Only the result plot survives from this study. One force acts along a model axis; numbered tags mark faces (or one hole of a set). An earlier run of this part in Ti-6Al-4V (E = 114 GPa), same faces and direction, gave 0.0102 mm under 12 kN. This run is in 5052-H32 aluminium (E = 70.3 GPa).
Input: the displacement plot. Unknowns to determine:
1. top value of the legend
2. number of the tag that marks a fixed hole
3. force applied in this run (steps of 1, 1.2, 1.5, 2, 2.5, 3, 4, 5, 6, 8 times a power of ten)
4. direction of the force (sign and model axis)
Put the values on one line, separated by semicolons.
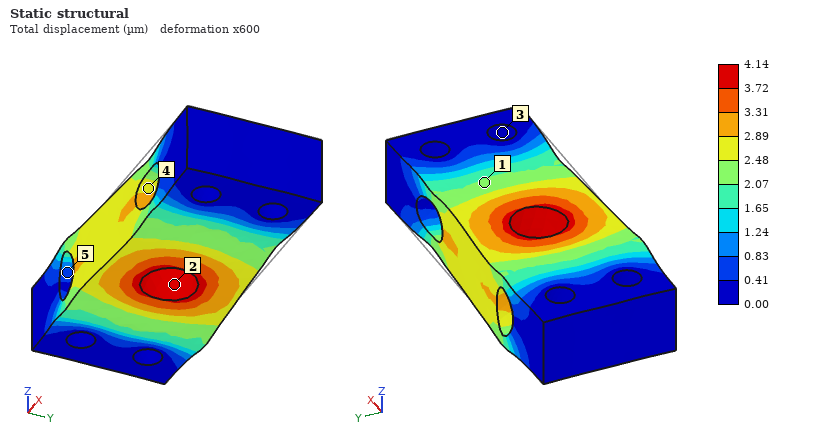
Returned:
4.14 µm; 3; 3 kN; -X
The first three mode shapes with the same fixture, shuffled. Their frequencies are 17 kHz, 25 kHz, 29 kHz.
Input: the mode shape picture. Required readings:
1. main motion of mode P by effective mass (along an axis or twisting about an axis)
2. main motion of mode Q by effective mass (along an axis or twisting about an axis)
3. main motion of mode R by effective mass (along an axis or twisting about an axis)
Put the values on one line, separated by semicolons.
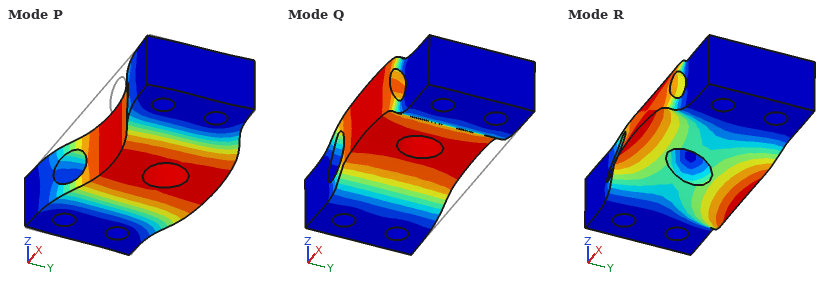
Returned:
along Y; along Z; twisting about X
